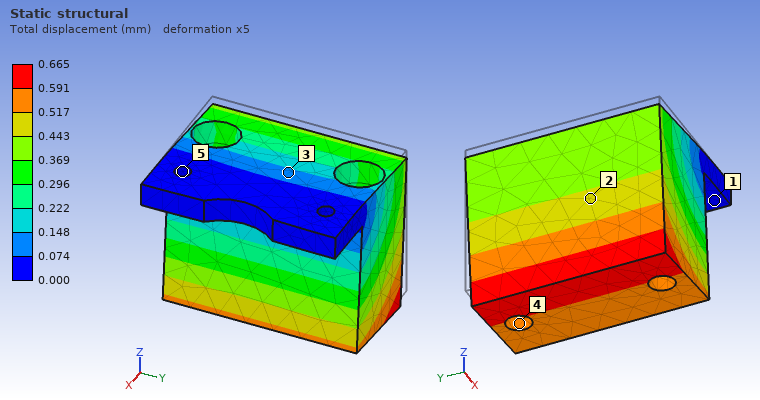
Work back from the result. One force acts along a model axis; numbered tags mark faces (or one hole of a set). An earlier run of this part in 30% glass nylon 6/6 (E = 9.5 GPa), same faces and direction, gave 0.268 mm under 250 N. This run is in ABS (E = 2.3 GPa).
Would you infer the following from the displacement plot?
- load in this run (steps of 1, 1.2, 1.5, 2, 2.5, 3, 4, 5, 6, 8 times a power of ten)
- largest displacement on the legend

150 N
0.665 mm
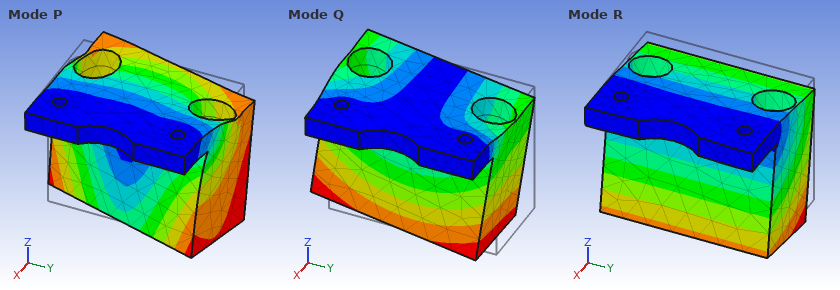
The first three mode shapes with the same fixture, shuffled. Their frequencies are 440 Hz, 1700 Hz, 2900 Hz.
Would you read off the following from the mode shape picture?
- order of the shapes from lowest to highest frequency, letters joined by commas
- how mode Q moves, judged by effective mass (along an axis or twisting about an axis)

R, Q, P
along Y
